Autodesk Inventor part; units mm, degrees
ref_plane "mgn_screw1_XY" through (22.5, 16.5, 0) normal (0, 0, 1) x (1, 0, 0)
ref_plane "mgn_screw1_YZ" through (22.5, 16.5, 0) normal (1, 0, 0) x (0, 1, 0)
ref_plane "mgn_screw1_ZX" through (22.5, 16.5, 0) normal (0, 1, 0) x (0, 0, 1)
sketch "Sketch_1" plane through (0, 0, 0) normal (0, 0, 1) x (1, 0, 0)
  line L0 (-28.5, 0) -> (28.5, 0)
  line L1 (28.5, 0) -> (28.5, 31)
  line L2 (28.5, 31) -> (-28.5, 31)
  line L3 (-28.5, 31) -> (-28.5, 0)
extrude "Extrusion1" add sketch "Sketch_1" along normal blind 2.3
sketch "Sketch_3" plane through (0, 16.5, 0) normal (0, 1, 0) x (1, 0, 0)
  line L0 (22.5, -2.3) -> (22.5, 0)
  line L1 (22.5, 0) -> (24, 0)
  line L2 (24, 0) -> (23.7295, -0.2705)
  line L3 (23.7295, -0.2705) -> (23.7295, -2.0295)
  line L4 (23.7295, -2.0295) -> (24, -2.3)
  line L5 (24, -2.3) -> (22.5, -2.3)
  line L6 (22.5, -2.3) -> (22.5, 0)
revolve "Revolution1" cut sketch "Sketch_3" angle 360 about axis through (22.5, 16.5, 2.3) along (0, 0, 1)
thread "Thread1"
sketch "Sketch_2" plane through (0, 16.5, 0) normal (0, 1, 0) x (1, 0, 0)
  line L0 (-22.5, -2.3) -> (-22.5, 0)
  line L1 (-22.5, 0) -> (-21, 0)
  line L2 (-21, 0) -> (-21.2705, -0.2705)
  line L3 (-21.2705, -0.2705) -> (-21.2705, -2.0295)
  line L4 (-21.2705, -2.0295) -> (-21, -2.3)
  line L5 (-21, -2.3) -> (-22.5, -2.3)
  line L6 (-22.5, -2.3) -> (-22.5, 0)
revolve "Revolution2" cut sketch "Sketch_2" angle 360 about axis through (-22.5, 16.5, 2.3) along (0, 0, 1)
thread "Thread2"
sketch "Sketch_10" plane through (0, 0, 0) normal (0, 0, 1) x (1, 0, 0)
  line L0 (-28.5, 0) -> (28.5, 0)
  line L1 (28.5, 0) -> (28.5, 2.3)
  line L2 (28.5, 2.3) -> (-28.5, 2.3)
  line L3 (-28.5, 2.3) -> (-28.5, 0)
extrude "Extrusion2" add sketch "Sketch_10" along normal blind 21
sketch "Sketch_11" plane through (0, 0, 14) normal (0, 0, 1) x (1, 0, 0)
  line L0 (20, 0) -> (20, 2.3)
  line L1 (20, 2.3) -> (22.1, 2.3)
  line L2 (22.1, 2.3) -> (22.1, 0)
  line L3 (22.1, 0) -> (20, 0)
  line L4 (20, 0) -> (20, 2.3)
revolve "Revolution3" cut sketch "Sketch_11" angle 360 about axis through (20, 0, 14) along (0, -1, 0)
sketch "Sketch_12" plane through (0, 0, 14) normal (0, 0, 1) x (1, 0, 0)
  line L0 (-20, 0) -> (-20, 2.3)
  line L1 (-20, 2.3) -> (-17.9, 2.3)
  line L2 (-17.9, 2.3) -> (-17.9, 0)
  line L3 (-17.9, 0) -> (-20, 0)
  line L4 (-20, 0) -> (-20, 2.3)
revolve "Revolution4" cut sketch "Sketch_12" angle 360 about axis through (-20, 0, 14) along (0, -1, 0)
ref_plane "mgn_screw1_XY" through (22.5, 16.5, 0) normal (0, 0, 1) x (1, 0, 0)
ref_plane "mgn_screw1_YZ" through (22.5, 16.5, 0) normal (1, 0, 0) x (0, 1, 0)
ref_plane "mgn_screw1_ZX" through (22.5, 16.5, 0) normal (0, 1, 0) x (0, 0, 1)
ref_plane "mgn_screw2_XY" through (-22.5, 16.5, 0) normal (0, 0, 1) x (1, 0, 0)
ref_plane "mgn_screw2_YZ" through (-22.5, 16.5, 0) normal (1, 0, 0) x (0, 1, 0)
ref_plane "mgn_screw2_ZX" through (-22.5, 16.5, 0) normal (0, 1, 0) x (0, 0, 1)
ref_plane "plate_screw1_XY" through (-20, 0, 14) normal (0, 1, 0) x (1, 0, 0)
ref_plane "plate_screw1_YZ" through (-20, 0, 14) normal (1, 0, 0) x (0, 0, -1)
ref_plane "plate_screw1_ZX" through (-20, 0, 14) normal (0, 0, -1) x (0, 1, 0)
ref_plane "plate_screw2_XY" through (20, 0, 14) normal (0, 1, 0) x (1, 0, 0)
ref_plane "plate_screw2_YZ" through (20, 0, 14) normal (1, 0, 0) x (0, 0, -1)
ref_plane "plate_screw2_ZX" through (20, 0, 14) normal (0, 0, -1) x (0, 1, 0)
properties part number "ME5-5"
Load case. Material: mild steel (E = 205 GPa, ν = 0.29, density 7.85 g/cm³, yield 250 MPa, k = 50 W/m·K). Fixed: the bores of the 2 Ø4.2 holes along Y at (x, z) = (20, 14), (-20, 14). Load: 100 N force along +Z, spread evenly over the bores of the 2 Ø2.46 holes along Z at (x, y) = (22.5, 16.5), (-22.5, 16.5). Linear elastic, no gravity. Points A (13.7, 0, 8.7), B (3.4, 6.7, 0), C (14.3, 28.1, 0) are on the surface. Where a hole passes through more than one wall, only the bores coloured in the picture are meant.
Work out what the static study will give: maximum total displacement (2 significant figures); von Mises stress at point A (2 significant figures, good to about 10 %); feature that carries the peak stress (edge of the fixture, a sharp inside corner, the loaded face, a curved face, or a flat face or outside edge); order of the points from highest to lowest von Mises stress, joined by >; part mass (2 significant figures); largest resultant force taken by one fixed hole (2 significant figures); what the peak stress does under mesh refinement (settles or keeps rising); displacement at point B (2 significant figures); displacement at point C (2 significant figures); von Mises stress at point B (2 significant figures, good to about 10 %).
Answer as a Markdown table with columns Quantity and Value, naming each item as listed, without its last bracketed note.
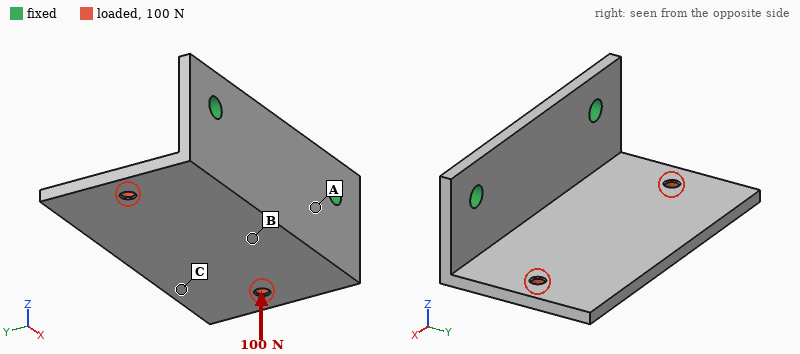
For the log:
| Quantity | Value |
|---|---|
| maximum total displacement | 78 µm |
| von Mises stress at point A | 27 MPa |
| feature that carries the peak stress | edge of the fixture |
| order of the points from highest to lowest von Mises stress, joined by > | A > B > C |
| part mass | 50 g |
| largest resultant force taken by one fixed hole | 50 N |
| what the peak stress does under mesh refinement | keeps rising |
| displacement at point B | 17 µm |
| displacement at point C | 65 µm |
| von Mises stress at point B | 16 MPa |
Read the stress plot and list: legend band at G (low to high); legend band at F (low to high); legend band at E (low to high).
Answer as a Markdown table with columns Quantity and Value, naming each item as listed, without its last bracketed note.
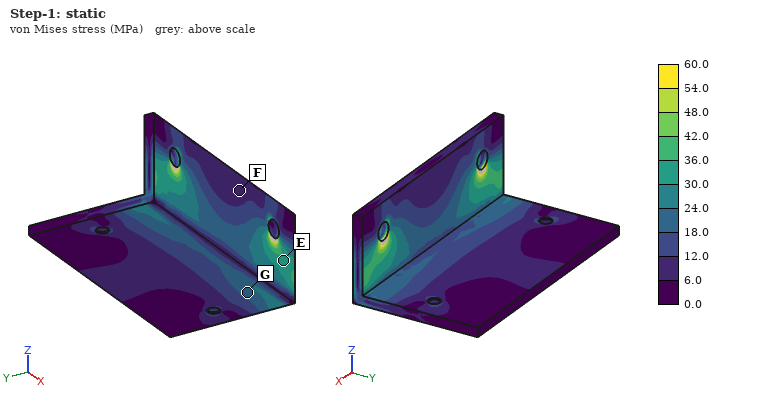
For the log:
| Quantity | Value |
|---|---|
| legend band at G | 18.0 to 24.0 MPa |
| legend band at F | 6.0 to 12.0 MPa |
| legend band at E | 30.0 to 36.0 MPa |
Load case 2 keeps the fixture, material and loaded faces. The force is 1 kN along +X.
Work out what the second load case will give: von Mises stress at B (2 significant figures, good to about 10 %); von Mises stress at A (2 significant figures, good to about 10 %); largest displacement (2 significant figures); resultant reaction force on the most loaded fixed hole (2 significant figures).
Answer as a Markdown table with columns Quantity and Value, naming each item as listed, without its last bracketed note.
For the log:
| Quantity | Value |
|---|---|
| von Mises stress at B | 20 MPa |
| von Mises stress at A | 58 MPa |
| largest displacement | 92 µm |
| resultant reaction force on the most loaded fixed hole | 680 N |
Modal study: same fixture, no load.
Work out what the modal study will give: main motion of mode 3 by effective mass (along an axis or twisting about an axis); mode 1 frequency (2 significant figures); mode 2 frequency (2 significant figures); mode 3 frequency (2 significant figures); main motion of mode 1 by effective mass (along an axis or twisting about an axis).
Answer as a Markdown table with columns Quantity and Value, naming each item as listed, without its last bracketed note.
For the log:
| Quantity | Value |
|---|---|
| main motion of mode 3 by effective mass | along X |
| mode 1 frequency | 1300 Hz |
| mode 2 frequency | 2500 Hz |
| mode 3 frequency | 4300 Hz |
| main motion of mode 1 by effective mass | along Z |
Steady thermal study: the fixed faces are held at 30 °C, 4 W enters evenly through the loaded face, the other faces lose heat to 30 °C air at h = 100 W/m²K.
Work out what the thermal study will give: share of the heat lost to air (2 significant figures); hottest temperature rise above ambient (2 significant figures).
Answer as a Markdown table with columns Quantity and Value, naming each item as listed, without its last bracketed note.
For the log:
| Quantity | Value |
|---|---|
| share of the heat lost to air | 69 % |
| hottest temperature rise above ambient | 14 K |
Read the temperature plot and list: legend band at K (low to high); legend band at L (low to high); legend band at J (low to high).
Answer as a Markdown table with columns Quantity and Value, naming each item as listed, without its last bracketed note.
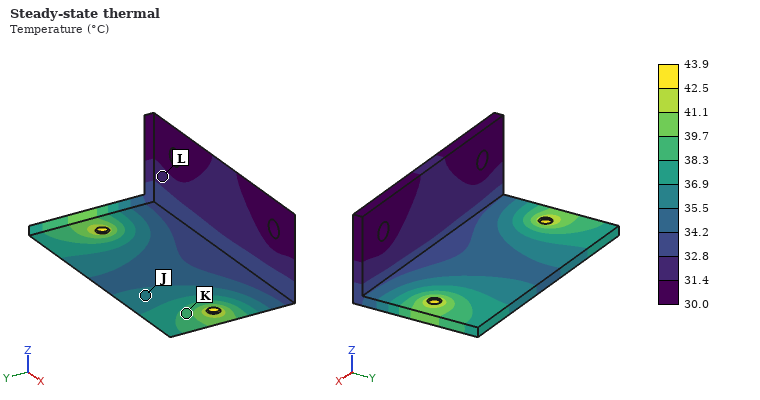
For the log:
| Quantity | Value |
|---|---|
| legend band at K | 38.3 to 39.7 °C |
| legend band at L | 31.4 to 32.8 °C |
| legend band at J | 35.5 to 36.9 °C |
